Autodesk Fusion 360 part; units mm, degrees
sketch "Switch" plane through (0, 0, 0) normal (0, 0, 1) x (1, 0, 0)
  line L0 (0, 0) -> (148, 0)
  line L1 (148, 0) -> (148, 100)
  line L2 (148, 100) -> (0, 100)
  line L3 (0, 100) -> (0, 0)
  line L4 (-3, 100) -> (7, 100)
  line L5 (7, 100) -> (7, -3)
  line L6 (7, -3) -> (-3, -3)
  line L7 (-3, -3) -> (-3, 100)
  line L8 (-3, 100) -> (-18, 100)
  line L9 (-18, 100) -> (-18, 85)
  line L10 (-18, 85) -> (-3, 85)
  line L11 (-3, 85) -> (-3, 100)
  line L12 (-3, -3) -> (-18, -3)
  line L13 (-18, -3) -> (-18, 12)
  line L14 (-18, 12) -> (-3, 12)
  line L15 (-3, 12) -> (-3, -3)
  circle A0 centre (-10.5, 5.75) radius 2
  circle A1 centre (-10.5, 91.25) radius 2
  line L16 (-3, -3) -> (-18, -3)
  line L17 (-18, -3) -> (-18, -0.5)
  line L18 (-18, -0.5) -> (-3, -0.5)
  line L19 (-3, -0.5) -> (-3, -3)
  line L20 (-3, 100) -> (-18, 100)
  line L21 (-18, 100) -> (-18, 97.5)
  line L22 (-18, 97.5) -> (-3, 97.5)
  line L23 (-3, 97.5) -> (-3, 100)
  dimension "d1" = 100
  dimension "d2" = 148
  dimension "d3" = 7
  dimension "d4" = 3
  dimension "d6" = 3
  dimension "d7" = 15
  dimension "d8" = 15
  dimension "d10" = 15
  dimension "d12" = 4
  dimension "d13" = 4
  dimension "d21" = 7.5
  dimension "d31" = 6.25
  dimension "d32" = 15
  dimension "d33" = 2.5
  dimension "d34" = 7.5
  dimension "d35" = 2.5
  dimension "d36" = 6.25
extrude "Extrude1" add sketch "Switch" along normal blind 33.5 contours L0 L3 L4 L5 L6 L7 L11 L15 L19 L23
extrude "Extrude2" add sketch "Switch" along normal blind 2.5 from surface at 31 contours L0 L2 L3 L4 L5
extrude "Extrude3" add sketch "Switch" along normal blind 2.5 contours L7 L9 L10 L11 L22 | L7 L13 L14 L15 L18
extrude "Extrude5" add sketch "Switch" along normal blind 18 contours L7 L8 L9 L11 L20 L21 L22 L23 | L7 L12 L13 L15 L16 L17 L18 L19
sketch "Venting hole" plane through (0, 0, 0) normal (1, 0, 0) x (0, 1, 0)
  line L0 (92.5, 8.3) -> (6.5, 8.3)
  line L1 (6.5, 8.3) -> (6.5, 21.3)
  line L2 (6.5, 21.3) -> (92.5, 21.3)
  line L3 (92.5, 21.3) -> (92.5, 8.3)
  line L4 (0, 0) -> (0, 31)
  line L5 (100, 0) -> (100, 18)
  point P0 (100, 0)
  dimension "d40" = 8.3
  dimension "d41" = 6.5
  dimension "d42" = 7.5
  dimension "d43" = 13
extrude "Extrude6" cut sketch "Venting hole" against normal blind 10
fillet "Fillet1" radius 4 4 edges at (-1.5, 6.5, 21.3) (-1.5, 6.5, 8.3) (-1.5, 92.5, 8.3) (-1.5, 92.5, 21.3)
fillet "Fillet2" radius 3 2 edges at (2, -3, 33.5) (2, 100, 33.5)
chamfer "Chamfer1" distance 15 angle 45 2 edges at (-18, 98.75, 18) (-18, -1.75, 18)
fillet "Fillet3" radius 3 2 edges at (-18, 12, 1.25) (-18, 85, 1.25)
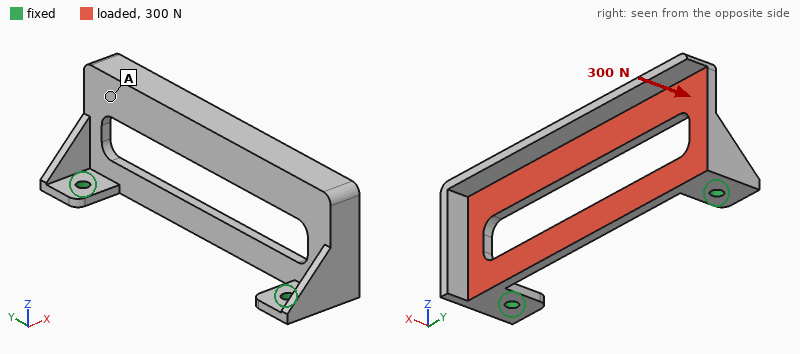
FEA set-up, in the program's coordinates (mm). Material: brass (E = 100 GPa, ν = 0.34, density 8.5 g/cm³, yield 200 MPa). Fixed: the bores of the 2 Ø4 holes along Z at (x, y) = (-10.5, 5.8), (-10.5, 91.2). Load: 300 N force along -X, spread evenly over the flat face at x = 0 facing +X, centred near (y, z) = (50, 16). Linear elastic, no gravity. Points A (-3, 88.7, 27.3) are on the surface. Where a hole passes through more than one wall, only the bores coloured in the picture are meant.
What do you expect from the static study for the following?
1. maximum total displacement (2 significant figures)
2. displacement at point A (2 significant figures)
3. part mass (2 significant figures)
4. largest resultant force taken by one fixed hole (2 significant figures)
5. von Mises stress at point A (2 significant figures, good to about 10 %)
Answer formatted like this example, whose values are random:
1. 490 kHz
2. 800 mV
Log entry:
1. 0.17 mm
2. 0.11 mm
3. 94 g
4. 160 N
5. 14 MPa
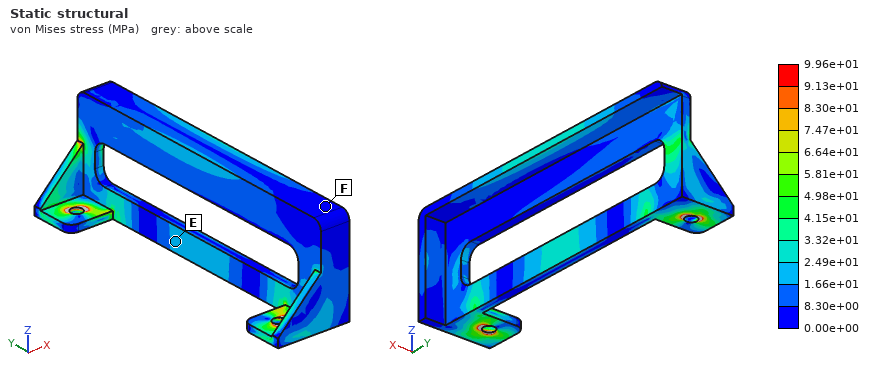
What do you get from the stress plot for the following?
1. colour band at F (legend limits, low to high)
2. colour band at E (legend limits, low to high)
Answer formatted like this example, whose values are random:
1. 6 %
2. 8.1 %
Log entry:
1. 0.00e+00 to 8.30e+00 MPa
2. 1.66e+01 to 2.49e+01 MPa
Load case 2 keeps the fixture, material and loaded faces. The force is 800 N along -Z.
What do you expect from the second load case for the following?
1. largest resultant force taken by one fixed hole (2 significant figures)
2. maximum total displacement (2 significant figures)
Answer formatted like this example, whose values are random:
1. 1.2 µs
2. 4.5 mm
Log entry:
1. 420 N
2. 0.21 mm
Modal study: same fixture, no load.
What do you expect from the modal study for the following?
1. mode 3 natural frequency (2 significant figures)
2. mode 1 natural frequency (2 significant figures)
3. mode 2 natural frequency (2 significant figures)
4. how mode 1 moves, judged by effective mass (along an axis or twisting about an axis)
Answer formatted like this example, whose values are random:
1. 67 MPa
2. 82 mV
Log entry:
1. 1600 Hz
2. 730 Hz
3. 1400 Hz
4. along X
